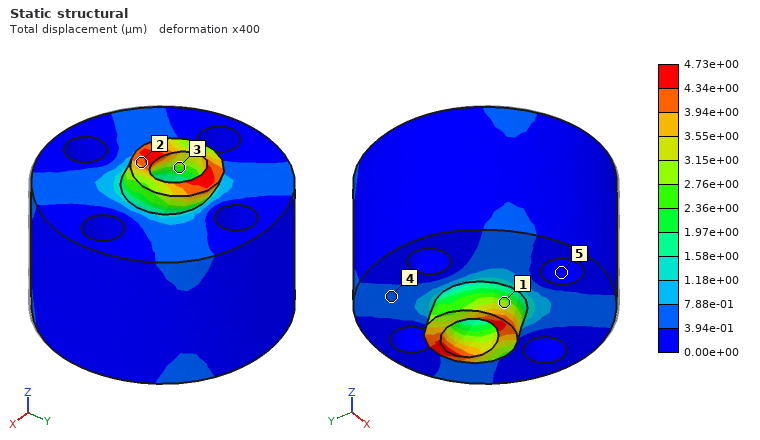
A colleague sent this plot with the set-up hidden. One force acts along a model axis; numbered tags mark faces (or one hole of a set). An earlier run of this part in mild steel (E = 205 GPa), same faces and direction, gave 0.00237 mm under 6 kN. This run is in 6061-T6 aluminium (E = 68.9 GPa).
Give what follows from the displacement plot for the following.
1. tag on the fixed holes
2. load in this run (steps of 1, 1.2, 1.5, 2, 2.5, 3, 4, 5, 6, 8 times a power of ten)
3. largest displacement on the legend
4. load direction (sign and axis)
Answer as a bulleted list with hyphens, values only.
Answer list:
- 5
- 4 kN
- 4.73e+00 µm
- +Y
